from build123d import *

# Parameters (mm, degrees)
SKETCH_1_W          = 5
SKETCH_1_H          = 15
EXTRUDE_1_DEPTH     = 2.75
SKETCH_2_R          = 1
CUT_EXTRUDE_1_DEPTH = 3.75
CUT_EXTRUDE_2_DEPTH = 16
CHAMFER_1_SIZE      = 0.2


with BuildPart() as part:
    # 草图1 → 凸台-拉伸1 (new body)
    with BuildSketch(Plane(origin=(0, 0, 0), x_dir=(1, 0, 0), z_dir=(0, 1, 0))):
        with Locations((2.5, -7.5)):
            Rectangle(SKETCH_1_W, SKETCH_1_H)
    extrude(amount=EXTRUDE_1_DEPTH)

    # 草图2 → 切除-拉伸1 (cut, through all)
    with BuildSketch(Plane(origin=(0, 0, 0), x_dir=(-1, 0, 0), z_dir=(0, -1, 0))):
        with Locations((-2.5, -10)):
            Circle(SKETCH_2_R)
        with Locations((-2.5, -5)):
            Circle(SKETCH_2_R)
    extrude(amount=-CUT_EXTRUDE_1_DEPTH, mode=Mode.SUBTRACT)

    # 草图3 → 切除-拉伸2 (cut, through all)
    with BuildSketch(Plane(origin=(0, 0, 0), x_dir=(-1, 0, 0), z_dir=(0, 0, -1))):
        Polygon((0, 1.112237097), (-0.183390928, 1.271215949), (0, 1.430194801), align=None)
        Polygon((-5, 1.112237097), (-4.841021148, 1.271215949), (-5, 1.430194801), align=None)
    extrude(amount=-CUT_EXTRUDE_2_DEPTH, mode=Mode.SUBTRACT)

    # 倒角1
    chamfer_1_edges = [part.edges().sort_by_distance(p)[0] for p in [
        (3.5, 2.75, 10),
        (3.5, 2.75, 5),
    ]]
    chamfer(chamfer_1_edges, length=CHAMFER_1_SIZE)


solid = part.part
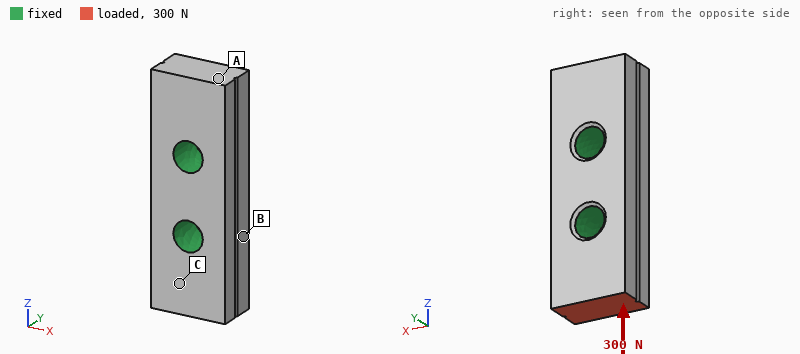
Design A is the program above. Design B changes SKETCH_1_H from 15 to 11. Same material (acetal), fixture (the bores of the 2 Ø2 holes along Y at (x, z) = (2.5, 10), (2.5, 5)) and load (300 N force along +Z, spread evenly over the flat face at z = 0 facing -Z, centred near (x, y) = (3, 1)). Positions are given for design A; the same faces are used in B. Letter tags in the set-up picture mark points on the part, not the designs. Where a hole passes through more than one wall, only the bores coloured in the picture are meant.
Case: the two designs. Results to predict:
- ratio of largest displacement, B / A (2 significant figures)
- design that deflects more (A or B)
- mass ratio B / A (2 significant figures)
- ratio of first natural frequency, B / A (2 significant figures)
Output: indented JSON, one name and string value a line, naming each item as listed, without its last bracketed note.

{
  "ratio of largest displacement, B / A": "0.77",
  "design that deflects more": "A",
  "mass ratio B / A": "0.71",
  "ratio of first natural frequency, B / A": "2.3"
}
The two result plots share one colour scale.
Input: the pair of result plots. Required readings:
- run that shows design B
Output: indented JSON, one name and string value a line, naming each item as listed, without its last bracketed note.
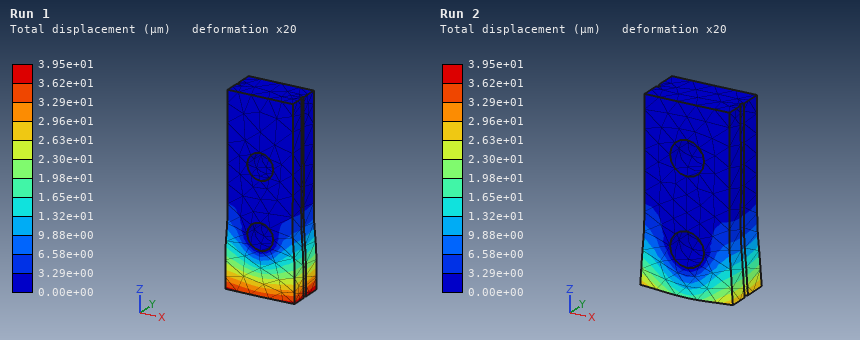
{
  "run that shows design B": "Run 2"
}
